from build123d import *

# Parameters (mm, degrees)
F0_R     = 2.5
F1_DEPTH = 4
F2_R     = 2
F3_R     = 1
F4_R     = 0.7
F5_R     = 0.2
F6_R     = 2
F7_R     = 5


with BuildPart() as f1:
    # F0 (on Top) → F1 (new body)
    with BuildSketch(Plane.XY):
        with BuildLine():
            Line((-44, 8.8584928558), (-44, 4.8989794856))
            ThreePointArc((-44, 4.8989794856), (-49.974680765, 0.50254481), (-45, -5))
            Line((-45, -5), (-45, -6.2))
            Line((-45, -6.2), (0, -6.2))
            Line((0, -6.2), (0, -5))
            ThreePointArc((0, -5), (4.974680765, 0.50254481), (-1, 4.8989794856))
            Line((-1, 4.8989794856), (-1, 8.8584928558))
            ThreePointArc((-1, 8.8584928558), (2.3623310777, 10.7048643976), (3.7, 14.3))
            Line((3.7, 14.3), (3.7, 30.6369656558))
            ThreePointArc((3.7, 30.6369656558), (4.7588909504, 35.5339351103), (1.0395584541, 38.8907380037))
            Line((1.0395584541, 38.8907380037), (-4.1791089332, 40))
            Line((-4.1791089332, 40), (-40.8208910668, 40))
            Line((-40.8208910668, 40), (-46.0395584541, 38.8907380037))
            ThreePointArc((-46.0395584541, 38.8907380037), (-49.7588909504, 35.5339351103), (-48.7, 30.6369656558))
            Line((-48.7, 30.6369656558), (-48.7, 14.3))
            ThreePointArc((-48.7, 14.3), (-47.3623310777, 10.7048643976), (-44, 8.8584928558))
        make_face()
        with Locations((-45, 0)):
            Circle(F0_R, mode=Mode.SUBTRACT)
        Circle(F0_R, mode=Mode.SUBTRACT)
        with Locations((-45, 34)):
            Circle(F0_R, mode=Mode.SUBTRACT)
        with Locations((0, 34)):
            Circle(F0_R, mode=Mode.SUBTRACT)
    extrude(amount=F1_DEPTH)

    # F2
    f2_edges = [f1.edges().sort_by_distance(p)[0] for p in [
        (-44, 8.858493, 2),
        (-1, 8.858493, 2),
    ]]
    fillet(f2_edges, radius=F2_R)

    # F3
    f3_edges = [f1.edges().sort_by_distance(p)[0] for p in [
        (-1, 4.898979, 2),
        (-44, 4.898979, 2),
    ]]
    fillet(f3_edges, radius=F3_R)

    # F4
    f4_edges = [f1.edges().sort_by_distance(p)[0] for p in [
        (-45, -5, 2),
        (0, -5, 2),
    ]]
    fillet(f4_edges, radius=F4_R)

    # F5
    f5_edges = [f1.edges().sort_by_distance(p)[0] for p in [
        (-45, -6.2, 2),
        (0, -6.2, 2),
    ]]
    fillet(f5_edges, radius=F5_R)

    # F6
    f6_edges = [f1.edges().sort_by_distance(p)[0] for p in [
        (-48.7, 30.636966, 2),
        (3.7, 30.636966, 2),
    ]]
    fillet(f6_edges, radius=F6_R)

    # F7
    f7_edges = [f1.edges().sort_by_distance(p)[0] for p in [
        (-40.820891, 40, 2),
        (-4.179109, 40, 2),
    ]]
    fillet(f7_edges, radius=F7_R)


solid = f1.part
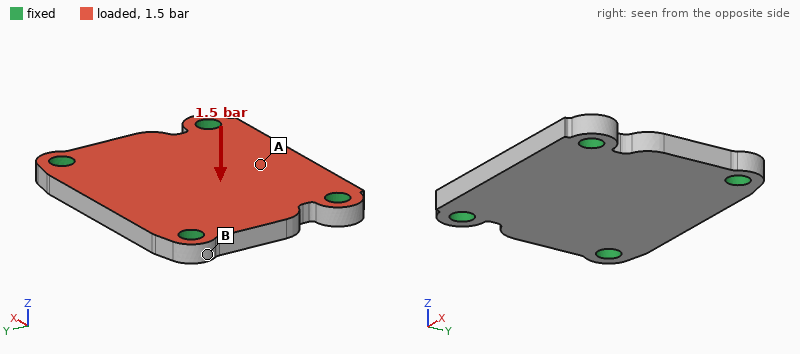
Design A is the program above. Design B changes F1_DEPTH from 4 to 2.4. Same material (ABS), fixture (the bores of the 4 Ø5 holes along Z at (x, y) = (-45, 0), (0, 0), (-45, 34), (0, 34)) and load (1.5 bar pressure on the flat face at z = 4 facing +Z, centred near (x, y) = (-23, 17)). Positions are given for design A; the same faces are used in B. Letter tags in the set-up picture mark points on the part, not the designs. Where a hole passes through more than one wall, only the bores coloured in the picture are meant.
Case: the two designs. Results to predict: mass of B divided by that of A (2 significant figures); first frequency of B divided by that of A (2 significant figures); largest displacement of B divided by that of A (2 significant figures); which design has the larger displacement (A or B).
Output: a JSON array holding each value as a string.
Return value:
["0.60", "0.64", "4.1", "B"]
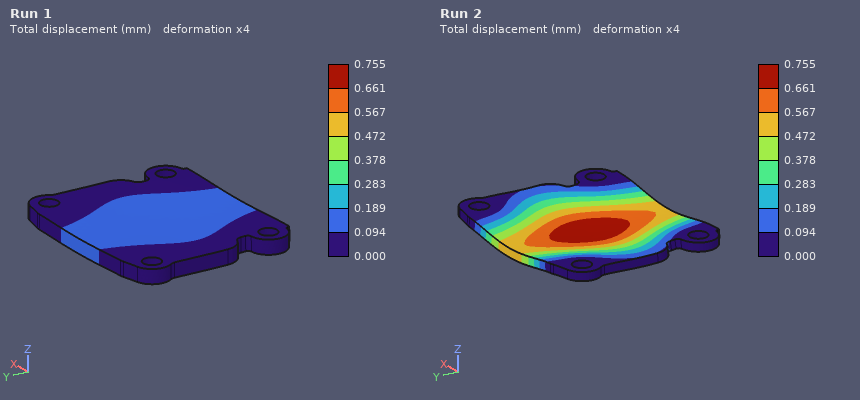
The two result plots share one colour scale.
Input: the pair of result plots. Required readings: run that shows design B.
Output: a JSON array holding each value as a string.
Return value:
["Run 2"]
